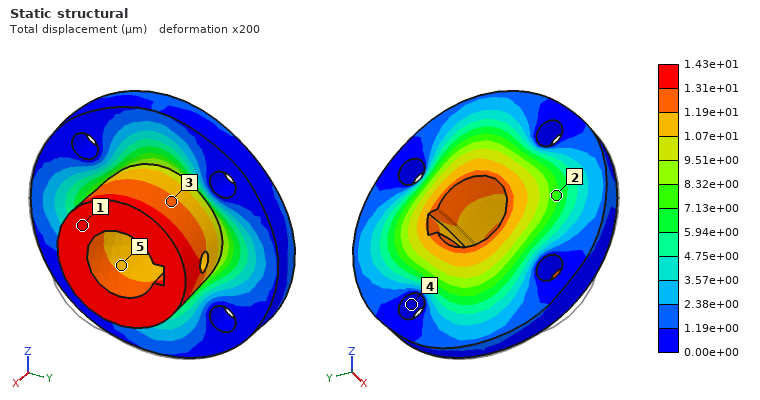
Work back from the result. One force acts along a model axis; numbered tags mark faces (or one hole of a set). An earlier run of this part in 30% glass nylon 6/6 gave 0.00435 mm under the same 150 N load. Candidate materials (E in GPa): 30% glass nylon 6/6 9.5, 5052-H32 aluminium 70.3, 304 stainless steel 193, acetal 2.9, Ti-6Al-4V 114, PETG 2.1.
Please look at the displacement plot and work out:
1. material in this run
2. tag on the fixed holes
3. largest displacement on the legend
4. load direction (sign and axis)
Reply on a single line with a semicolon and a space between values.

acetal; 4; 1.43e+01 µm; -X
